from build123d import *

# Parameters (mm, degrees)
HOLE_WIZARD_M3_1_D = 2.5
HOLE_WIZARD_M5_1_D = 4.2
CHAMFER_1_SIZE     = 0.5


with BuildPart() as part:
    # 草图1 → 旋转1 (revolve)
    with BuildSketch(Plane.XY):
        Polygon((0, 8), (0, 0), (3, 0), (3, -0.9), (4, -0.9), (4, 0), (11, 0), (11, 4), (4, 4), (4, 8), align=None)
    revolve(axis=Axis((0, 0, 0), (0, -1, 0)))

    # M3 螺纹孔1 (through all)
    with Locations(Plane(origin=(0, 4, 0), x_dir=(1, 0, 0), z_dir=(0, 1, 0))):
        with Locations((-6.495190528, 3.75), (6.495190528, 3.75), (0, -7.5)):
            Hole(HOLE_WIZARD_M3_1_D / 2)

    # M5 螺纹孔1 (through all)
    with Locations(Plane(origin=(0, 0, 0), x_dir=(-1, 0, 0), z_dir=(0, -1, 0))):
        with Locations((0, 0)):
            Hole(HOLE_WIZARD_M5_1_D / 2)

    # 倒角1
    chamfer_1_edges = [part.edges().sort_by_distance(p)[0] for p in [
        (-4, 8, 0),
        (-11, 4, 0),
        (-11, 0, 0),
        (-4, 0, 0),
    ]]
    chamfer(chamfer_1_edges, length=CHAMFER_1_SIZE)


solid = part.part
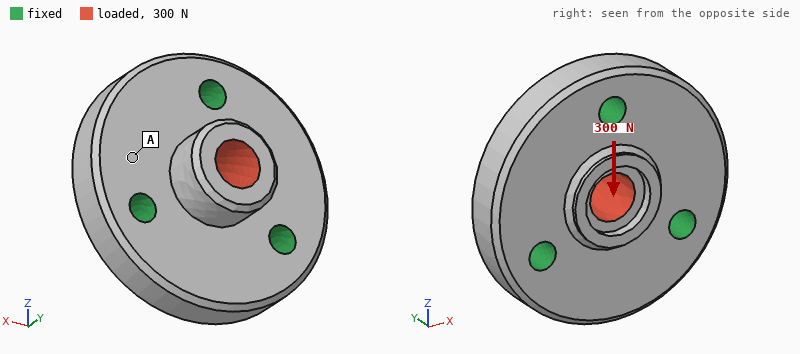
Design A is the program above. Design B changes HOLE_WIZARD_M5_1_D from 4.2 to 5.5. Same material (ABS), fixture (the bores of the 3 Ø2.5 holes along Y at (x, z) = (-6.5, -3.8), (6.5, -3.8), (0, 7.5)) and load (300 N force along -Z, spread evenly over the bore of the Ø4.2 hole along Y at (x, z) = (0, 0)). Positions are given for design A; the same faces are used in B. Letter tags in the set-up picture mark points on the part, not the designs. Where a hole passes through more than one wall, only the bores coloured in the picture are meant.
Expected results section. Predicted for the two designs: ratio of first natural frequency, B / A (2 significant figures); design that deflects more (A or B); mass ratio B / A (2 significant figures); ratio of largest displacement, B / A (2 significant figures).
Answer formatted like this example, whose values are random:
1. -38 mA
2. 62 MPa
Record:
1. 0.99
2. B
3. 0.95
4. 1.3
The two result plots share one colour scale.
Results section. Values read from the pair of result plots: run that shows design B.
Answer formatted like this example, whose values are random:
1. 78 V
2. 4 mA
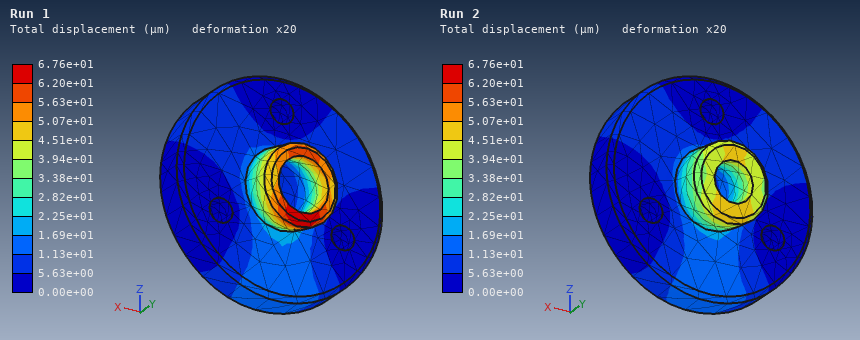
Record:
1. Run 1
